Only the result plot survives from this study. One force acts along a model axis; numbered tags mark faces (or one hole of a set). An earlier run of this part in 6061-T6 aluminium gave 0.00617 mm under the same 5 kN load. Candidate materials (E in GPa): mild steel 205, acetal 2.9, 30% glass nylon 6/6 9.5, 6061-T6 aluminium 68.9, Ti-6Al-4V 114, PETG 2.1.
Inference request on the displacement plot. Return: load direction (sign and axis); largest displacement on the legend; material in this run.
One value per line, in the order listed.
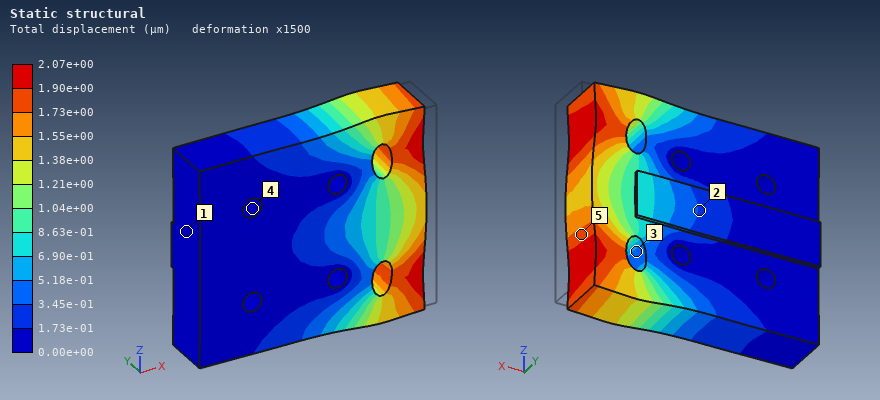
-X
2.07e+00 µm
mild steel
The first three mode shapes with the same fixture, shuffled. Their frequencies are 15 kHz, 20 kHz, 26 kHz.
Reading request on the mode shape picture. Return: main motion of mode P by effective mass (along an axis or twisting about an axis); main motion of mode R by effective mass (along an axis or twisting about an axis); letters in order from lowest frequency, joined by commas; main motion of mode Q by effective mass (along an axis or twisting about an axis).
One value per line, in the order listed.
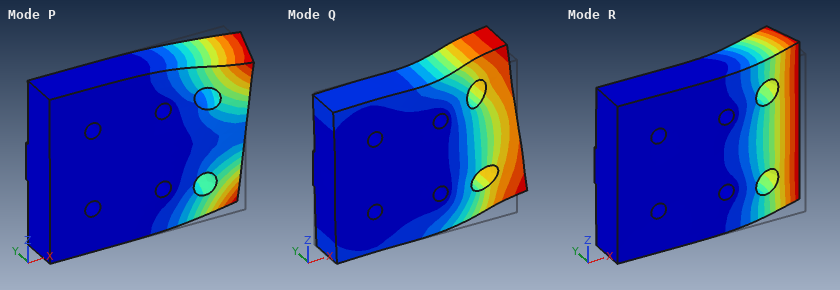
twisting about X
along Y
R, P, Q
along Z
